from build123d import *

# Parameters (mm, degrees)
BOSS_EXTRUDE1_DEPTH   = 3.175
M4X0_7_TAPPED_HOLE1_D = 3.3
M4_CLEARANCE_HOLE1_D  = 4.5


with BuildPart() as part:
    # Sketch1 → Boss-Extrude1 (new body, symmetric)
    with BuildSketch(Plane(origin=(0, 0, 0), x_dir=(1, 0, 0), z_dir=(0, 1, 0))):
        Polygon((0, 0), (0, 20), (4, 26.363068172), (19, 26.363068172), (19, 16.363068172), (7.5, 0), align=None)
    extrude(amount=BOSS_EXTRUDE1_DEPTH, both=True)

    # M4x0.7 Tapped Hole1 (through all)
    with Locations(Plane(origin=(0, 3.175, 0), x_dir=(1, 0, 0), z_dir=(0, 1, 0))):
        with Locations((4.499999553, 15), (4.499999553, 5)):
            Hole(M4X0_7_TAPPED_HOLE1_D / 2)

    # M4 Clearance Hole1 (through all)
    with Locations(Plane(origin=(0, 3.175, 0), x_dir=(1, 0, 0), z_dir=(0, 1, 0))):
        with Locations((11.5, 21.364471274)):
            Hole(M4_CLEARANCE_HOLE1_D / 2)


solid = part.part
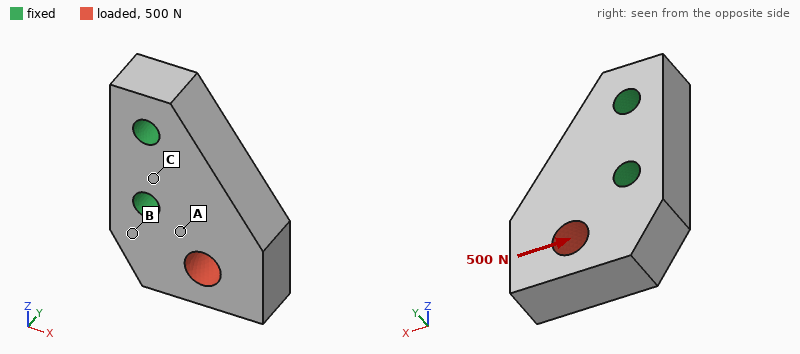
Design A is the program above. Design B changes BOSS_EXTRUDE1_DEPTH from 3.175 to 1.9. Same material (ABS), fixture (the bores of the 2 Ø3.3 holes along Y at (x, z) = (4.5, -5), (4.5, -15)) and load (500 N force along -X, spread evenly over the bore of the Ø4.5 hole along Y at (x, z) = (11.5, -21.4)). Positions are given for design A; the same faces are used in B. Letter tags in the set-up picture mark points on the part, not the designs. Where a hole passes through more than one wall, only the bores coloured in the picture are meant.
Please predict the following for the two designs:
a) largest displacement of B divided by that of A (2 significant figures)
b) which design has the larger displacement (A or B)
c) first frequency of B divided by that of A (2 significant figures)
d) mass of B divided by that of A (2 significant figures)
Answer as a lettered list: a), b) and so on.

a) 1.7
b) B
c) 0.69
d) 0.60
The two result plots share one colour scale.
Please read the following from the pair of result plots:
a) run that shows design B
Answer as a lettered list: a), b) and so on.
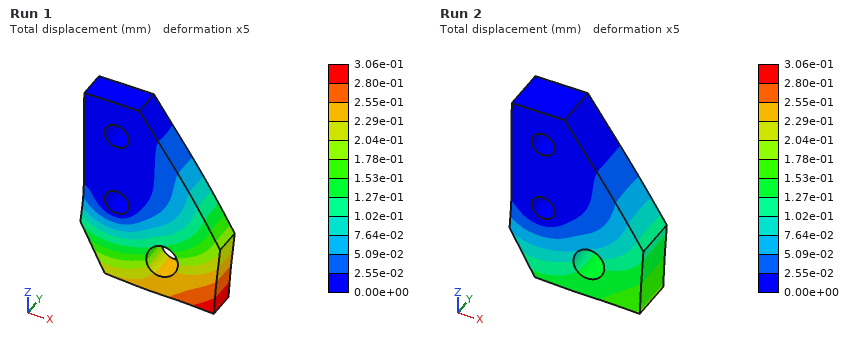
a) Run 1
